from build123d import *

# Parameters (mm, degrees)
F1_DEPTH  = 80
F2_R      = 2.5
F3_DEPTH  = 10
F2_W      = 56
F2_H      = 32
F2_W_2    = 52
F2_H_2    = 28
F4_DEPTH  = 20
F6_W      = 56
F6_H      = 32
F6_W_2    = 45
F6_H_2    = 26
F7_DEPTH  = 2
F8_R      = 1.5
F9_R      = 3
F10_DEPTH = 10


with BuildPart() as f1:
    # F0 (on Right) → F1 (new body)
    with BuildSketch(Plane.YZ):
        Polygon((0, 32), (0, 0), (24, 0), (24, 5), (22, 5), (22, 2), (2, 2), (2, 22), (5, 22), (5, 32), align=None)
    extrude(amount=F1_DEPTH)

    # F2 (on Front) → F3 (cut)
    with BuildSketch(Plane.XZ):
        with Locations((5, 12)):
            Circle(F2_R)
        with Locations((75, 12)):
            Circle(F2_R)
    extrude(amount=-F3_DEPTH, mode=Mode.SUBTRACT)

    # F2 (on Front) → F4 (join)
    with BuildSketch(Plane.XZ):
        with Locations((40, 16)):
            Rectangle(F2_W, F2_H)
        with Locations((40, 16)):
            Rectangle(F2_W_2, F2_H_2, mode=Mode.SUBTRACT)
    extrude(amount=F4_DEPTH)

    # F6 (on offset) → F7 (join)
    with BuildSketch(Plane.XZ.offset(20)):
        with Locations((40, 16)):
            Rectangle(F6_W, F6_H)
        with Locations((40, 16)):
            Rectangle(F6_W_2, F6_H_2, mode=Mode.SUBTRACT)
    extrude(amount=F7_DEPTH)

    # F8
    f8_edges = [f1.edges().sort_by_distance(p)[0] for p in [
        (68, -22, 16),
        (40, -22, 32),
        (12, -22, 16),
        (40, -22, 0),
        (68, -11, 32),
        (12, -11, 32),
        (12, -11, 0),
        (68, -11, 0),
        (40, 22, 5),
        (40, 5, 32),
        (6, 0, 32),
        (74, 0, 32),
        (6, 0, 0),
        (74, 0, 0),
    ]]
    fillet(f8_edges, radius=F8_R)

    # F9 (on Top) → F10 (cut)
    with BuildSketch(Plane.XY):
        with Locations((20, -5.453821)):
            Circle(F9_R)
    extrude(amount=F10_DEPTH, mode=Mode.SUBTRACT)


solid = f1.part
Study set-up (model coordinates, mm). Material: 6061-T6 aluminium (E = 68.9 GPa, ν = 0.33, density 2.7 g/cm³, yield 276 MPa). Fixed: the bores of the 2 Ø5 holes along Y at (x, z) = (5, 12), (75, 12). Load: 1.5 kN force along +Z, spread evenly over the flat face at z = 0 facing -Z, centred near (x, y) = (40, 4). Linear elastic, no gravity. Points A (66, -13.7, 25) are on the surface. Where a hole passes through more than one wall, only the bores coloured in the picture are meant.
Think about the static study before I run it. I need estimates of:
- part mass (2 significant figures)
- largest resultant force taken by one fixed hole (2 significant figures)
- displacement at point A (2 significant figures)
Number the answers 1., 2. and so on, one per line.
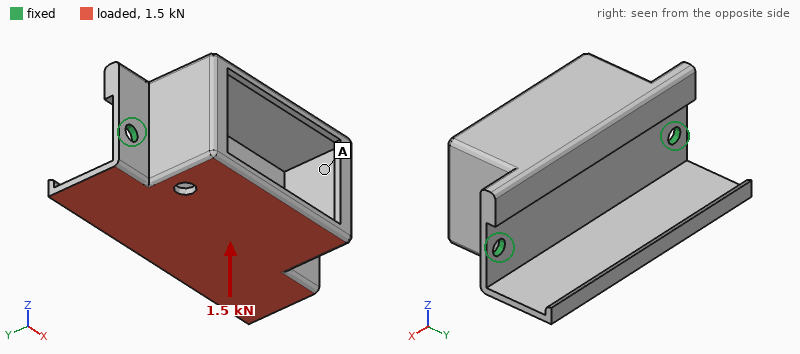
1. 52 g
2. 760 N
3. 0.089 mm
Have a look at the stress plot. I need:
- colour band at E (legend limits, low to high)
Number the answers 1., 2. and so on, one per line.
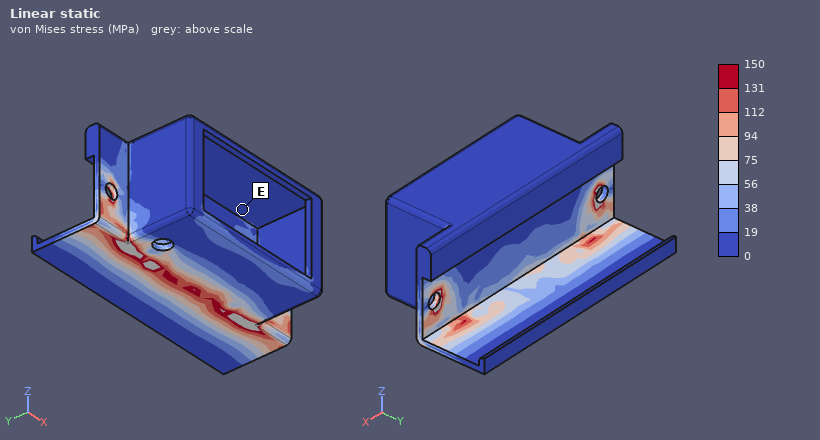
1. 0 to 19 MPa
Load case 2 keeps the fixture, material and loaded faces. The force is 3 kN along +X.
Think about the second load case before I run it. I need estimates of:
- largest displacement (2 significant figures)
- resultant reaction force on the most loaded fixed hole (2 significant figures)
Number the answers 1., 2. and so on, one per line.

1. 48 µm
2. 1.6 kN
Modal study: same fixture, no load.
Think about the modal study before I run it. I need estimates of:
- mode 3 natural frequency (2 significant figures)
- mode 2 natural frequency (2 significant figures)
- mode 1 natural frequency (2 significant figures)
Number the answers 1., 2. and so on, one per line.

1. 2700 Hz
2. 2700 Hz
3. 1400 Hz
